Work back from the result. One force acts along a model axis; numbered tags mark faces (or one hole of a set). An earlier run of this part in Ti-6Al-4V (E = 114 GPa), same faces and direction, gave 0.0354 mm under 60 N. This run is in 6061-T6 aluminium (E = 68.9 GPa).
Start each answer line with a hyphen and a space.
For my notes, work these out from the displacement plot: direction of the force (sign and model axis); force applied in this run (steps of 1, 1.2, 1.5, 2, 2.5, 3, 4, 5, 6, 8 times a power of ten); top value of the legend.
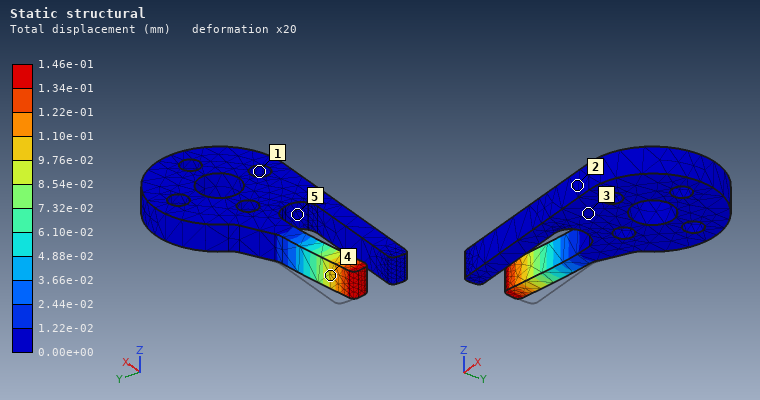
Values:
- -Y
- 150 N
- 1.46e-01 mm
